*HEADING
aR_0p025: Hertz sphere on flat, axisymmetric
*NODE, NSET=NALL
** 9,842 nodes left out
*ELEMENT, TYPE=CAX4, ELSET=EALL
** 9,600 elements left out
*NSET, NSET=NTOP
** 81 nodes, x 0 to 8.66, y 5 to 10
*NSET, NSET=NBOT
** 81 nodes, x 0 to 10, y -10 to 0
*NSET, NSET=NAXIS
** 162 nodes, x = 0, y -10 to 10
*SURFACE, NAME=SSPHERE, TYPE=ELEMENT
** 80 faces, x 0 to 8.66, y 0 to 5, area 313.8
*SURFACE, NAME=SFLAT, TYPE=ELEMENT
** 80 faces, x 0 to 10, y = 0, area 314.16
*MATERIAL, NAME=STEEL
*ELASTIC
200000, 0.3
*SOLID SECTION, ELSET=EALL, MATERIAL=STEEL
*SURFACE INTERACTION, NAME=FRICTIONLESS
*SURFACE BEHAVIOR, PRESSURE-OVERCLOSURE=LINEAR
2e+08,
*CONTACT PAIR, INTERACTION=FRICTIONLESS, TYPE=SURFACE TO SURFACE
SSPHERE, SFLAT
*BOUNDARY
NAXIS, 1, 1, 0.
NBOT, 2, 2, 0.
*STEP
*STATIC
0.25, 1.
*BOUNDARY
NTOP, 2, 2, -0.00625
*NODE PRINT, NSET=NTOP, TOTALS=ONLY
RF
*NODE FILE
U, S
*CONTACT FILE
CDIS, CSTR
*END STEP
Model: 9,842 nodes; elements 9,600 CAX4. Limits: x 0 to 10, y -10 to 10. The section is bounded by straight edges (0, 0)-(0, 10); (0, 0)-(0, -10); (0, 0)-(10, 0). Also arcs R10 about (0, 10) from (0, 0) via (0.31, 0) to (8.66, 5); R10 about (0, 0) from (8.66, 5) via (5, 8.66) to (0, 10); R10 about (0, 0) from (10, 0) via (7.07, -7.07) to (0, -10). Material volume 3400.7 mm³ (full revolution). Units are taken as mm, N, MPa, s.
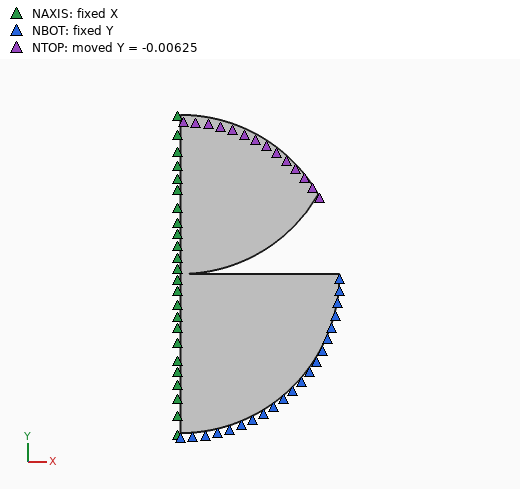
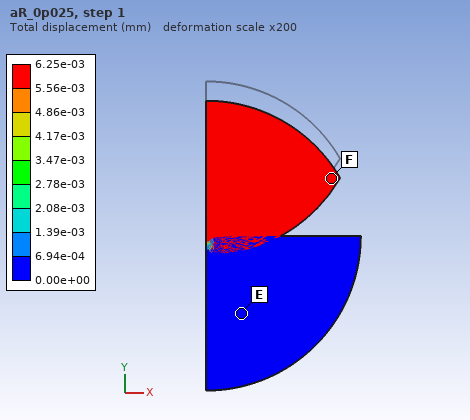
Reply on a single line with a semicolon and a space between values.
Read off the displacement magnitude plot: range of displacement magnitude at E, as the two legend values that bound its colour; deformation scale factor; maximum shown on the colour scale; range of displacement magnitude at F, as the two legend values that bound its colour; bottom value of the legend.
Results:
0.00e+00 to 6.94e-04 mm; 200; 6.25e-03 mm; 5.56e-03 to 6.25e-03 mm; 0.00e+00 mm
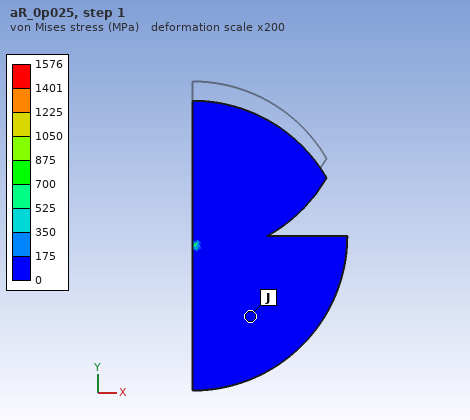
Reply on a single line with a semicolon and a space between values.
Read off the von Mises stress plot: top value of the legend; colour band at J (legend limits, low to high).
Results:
1576 MPa; 0 to 175 MPa
